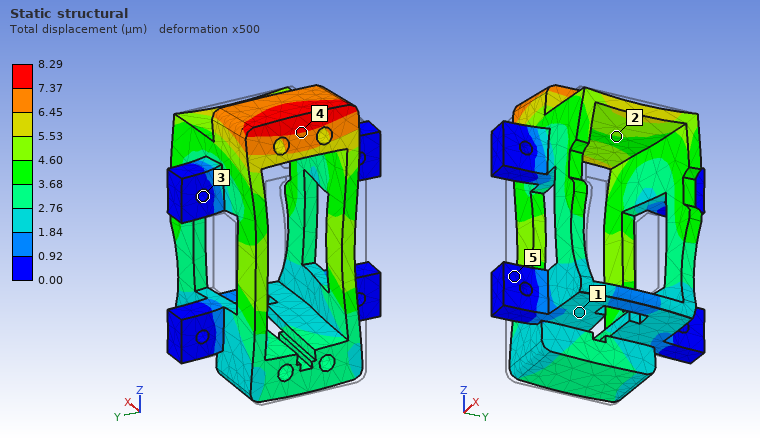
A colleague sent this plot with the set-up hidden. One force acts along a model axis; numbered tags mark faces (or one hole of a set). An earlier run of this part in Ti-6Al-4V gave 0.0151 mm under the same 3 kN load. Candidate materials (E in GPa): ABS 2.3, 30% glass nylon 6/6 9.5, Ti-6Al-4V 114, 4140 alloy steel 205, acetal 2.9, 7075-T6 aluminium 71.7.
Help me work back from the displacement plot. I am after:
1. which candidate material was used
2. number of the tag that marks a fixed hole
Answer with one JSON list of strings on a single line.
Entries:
["4140 alloy steel", "3"]
